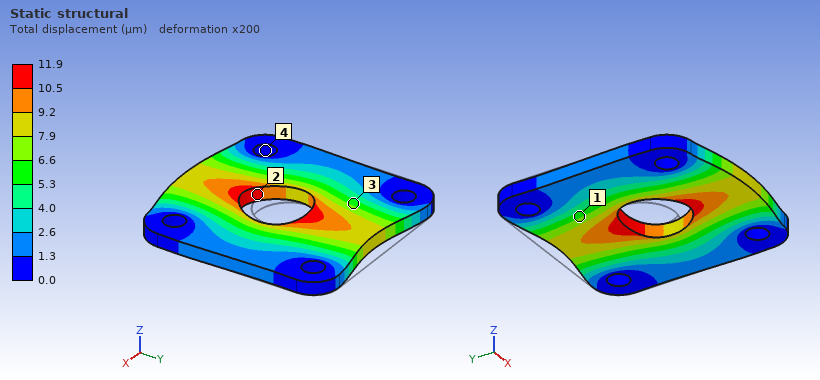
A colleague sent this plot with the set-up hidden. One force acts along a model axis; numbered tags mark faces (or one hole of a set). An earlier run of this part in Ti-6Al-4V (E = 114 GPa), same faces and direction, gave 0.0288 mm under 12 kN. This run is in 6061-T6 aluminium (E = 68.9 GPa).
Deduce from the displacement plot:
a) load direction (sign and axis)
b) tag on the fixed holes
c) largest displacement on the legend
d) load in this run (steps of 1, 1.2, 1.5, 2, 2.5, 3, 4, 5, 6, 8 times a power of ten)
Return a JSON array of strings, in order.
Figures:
["-Y", "4", "11.9 µm", "3 kN"]
